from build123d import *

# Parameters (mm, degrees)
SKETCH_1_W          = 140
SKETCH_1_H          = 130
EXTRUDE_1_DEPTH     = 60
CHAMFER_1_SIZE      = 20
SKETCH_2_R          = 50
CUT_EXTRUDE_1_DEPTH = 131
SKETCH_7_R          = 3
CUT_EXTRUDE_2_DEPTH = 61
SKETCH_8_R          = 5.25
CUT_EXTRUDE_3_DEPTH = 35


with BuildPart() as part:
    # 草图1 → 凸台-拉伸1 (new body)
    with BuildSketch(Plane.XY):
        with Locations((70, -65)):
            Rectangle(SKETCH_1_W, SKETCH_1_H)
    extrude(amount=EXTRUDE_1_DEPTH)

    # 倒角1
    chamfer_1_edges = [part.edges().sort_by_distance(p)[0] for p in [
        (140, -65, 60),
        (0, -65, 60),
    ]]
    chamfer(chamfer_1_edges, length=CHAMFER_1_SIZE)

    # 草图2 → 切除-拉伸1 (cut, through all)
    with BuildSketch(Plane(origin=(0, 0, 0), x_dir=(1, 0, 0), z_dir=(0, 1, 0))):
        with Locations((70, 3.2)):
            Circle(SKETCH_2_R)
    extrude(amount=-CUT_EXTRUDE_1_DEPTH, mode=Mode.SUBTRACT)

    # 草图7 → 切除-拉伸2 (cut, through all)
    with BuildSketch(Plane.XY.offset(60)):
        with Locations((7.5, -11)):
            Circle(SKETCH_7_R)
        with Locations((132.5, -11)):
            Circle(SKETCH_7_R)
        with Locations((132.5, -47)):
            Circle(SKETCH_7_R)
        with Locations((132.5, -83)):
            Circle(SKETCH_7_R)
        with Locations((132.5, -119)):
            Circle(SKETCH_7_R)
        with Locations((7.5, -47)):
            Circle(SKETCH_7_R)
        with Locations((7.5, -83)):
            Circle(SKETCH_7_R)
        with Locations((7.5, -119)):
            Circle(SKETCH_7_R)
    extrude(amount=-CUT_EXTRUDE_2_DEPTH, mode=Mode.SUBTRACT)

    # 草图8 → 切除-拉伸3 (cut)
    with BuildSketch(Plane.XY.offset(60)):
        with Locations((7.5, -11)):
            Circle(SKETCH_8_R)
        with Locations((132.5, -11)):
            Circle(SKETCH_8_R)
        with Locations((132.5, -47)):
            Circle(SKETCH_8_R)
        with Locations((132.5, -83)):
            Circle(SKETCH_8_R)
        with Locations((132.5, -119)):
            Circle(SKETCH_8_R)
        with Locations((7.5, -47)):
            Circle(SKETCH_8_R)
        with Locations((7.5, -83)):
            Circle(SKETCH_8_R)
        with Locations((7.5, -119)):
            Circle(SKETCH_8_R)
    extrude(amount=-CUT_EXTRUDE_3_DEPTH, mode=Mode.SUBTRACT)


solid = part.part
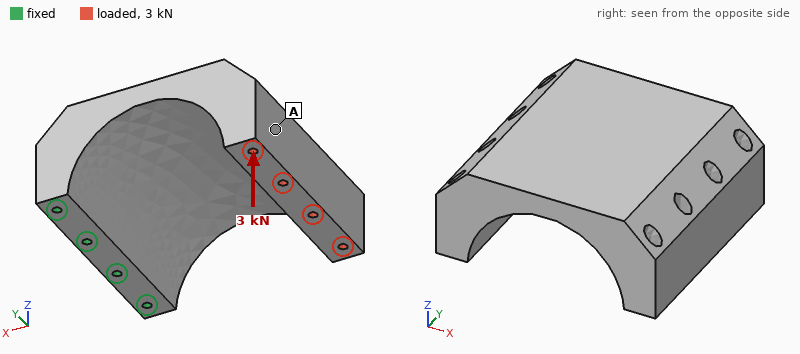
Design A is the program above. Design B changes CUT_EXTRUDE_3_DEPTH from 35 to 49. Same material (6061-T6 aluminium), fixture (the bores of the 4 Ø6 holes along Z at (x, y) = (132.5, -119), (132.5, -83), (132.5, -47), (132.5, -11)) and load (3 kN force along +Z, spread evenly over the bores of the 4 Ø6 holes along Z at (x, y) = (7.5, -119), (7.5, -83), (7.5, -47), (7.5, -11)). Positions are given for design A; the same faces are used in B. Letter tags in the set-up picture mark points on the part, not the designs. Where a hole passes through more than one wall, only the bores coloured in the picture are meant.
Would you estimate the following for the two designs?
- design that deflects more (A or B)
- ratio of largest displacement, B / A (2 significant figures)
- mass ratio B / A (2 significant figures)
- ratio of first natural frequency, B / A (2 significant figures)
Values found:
B
1.5
0.99
0.76
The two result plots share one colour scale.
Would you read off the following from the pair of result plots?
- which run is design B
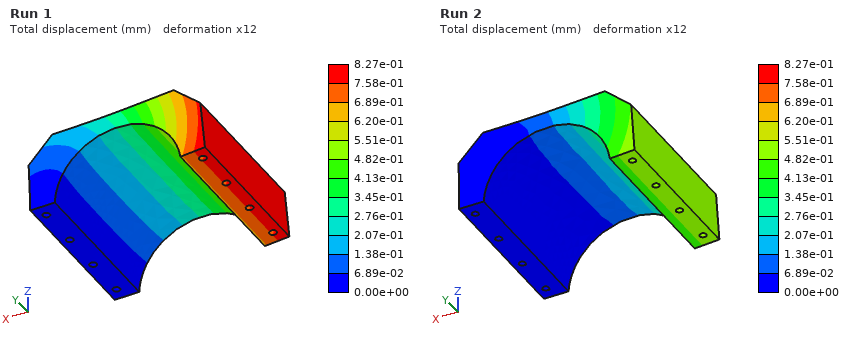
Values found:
Run 1
